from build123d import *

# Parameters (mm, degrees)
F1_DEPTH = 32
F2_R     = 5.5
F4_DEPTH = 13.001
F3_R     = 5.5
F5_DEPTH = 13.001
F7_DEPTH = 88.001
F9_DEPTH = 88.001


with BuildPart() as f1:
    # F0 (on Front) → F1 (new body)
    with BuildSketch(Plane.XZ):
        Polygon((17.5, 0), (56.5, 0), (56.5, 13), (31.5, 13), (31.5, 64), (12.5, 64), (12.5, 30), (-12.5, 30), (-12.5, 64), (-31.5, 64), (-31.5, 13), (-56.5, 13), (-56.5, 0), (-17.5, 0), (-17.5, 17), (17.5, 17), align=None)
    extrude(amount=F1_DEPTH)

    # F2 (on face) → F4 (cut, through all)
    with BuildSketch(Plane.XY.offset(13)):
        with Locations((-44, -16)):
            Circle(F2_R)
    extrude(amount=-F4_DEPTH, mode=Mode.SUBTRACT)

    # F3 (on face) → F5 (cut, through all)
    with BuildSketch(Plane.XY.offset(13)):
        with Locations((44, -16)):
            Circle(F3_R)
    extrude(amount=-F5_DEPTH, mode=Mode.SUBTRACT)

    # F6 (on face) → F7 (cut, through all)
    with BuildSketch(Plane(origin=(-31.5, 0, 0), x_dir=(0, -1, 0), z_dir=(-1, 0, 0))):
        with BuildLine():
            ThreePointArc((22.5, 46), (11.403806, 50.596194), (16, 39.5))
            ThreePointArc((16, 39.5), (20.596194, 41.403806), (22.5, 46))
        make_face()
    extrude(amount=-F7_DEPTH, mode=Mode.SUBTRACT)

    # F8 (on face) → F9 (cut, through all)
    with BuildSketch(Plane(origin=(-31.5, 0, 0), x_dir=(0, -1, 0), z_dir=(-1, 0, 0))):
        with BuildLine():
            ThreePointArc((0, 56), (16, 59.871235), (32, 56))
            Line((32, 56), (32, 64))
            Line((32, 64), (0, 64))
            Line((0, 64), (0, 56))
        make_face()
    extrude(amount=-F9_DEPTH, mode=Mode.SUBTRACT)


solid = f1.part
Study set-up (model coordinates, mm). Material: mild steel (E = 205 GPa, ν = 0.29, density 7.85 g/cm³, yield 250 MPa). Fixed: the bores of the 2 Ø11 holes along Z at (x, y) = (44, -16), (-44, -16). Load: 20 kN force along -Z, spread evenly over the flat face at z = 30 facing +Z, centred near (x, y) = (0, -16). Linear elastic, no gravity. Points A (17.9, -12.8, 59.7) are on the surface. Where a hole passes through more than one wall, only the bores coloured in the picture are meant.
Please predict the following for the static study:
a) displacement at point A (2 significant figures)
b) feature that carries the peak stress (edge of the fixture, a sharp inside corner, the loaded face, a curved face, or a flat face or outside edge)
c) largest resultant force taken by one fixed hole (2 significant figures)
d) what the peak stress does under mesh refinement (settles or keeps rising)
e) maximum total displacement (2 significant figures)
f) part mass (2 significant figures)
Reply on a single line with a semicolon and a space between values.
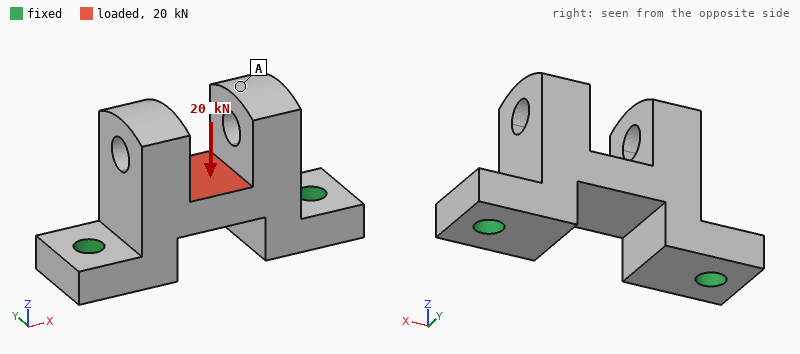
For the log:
28 µm; edge of the fixture; 15 kN; keeps rising; 30 µm; 700 g
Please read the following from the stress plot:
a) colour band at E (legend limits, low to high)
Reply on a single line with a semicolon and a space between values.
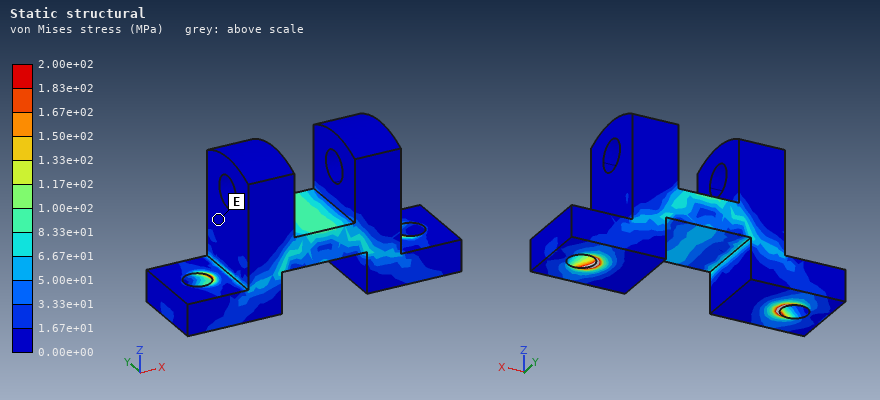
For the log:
0.00e+00 to 1.67e+01 MPa
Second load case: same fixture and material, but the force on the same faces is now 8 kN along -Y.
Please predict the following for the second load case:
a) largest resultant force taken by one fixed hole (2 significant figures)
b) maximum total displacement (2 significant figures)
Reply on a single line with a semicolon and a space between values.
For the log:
4.0 kN; 54 µm
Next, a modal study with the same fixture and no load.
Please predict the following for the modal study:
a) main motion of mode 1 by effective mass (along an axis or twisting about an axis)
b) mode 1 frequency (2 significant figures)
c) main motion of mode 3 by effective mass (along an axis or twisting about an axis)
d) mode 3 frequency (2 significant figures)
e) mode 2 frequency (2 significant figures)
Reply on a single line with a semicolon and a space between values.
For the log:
along Y; 3200 Hz; along X; 6700 Hz; 5400 Hz
